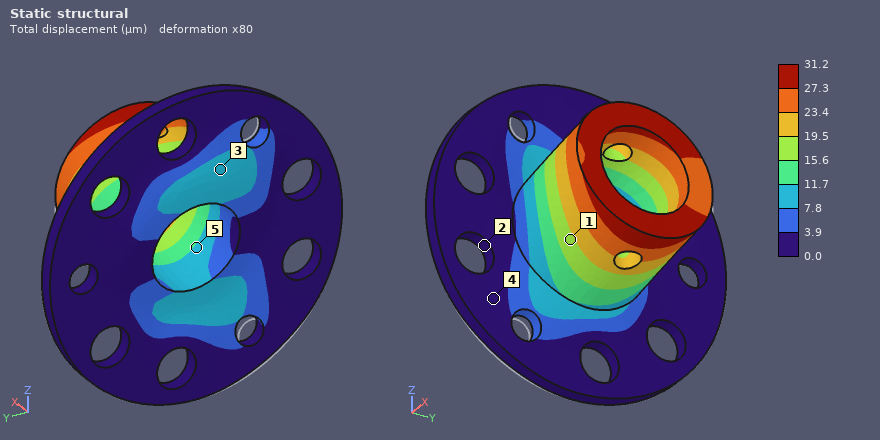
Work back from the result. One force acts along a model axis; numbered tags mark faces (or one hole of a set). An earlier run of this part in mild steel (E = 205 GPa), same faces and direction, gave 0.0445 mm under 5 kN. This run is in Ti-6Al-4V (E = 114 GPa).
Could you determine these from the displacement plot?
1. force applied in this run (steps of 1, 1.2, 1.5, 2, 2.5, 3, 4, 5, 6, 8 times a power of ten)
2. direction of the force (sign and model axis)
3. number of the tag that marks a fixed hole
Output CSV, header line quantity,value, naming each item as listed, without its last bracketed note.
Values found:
quantity,value
force applied in this run,2 kN
direction of the force,+Z
number of the tag that marks a fixed hole,2
